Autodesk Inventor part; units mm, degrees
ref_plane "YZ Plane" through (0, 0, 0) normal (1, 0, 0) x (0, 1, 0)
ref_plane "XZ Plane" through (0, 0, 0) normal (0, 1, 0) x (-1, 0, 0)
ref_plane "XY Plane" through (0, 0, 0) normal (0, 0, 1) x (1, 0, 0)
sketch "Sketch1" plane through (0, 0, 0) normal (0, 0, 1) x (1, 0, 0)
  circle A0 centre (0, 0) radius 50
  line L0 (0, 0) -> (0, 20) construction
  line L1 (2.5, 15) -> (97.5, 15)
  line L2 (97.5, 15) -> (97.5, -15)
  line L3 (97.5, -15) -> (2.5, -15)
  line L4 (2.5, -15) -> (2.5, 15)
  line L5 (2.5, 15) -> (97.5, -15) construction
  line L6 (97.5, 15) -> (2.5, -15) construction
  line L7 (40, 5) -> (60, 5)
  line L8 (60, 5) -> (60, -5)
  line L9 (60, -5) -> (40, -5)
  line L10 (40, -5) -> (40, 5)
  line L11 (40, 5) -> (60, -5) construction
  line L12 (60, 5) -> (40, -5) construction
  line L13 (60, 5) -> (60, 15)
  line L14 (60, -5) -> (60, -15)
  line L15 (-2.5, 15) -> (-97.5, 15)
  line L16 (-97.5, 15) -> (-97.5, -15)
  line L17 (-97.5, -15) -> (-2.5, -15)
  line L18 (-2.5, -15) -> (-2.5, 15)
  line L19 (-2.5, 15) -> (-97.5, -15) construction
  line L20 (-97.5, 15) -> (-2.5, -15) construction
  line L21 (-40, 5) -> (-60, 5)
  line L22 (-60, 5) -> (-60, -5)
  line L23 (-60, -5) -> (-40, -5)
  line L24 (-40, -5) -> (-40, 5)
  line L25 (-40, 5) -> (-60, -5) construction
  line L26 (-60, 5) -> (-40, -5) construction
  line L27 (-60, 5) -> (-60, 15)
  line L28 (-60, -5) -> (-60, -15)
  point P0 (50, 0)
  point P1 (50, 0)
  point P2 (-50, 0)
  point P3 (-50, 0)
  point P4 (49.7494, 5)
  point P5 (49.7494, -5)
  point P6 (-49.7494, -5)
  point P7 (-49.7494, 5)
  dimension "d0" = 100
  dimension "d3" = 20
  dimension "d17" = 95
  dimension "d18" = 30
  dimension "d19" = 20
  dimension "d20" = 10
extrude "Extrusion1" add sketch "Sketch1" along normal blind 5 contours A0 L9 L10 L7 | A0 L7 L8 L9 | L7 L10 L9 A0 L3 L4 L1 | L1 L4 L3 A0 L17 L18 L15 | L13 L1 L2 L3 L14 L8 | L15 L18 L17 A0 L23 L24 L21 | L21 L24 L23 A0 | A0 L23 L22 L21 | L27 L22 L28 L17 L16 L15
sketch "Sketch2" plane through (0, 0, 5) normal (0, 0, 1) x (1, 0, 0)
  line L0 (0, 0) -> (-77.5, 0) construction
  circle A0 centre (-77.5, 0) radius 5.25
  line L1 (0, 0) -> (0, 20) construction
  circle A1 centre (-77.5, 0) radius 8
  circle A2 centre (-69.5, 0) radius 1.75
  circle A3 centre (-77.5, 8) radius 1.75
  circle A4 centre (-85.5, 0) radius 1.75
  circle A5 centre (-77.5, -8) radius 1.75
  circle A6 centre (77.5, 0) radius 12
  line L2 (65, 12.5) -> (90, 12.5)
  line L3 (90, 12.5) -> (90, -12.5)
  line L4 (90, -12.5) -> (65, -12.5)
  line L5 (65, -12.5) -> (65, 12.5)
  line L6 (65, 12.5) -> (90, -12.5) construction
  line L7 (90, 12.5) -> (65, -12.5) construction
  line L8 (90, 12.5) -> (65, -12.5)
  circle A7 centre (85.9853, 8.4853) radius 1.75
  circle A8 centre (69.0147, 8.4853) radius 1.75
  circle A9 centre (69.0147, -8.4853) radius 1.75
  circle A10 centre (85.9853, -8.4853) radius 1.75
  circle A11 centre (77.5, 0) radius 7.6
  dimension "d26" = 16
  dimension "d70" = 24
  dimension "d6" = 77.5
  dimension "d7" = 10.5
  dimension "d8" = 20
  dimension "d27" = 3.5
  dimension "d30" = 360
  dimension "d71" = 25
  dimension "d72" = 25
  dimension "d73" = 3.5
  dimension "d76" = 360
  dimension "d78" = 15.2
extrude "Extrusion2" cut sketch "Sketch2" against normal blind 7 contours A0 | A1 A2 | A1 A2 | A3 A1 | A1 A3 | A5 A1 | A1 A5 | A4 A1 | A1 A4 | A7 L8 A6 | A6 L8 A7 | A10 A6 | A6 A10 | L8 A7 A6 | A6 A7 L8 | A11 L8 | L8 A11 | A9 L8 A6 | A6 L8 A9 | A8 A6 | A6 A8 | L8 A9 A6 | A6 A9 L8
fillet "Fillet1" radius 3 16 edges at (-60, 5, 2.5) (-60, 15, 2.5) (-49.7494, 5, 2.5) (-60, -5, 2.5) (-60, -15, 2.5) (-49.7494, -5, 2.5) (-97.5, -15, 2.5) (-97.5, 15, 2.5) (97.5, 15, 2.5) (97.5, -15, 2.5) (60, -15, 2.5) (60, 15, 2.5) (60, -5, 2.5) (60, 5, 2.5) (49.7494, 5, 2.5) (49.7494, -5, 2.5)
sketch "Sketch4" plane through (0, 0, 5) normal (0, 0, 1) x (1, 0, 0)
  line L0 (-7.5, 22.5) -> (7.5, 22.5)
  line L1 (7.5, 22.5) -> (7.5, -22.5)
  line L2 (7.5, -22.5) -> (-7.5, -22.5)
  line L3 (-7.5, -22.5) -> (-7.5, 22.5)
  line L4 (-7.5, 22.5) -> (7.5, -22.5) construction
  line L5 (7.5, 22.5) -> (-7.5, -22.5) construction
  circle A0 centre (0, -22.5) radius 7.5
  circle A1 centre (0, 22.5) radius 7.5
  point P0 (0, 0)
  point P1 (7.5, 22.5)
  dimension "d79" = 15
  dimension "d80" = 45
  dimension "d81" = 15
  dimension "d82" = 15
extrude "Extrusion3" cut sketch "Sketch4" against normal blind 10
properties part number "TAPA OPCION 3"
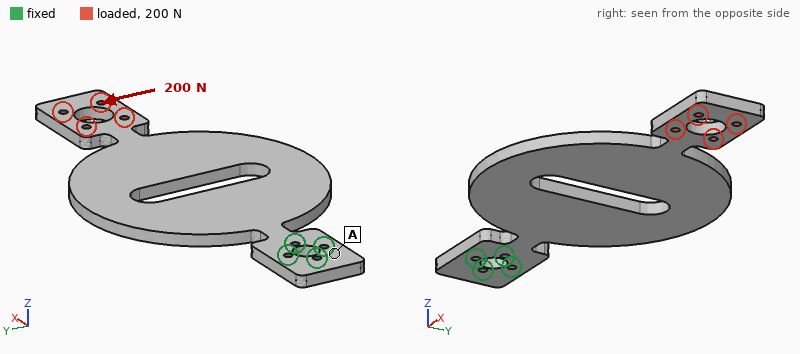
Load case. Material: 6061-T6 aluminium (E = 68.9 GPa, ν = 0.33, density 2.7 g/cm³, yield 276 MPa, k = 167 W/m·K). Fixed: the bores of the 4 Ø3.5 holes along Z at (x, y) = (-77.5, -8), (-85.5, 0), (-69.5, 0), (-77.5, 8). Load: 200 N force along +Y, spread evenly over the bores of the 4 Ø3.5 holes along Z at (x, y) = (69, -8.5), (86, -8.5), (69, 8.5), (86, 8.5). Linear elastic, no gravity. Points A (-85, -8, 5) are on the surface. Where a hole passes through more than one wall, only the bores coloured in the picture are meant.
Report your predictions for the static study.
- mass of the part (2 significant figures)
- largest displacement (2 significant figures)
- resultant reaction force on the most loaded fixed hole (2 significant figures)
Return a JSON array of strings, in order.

["120 g", "2.3 mm", "1.4 kN"]
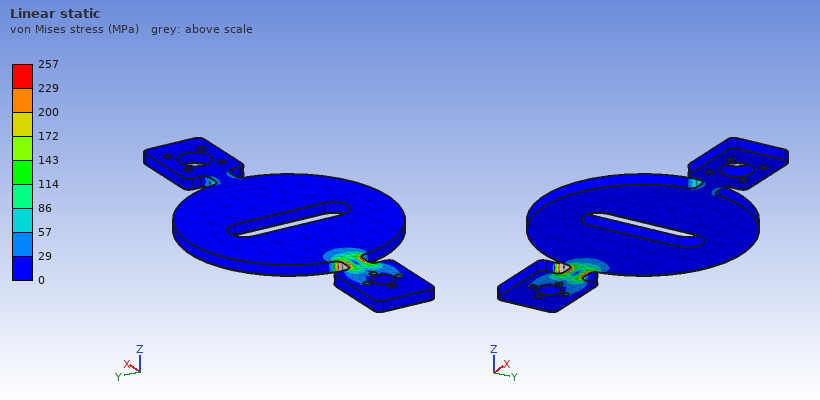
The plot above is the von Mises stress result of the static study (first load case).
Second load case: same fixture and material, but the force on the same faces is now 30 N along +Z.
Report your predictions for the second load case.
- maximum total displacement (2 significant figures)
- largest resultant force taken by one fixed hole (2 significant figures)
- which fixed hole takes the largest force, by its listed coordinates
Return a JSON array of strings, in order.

["2.4 mm", "250 N", "(-69.5, 0)"]
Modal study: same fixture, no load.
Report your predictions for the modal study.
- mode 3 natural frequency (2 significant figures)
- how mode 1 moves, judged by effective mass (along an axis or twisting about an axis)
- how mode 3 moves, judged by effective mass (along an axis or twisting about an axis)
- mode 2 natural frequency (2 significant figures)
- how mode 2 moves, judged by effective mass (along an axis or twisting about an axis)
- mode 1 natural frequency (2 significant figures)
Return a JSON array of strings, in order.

["370 Hz", "along Z", "twisting about X", "270 Hz", "along Y", "110 Hz"]
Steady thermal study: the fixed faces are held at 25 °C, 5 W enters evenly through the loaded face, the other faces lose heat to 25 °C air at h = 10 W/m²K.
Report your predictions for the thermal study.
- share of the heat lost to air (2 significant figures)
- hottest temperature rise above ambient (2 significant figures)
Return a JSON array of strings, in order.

["48 %", "28 K"]
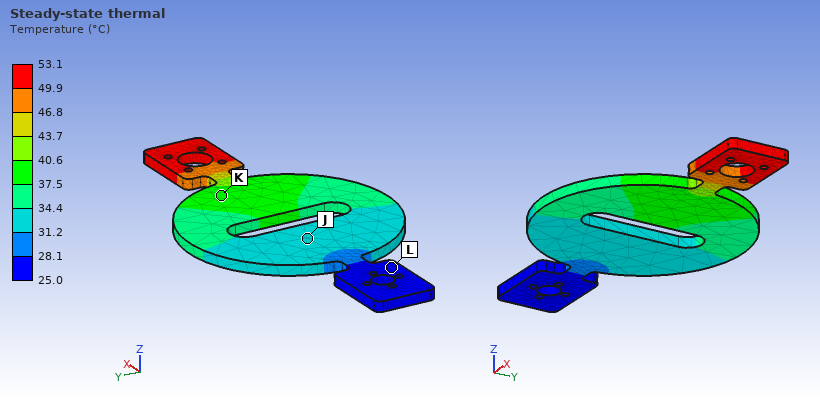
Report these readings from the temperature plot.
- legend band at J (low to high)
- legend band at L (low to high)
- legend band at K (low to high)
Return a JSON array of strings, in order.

["31.2 to 34.4 °C", "25.0 to 28.1 °C", "37.5 to 40.6 °C"]
